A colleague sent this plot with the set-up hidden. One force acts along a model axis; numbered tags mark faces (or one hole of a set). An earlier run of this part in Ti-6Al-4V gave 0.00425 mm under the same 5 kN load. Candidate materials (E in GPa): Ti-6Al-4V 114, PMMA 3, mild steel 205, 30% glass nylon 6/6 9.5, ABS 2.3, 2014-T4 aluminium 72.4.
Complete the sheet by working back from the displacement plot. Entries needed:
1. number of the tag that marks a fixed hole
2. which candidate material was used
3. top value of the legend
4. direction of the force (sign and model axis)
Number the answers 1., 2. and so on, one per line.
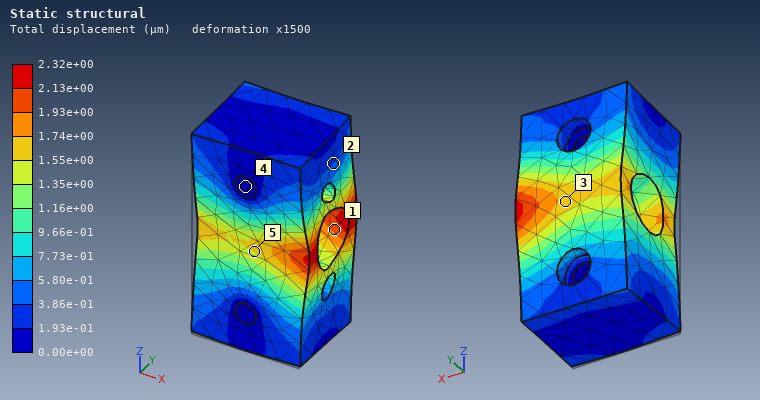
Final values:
1. 4
2. mild steel
3. 2.32e+00 µm
4. +Y
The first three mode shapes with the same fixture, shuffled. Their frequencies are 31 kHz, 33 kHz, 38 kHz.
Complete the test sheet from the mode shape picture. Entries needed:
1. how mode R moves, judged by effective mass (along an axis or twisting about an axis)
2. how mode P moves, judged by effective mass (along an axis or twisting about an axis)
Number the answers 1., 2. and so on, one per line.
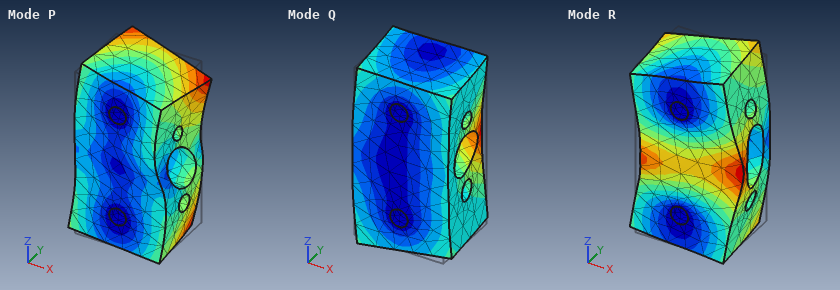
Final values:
1. twisting about Z
2. twisting about Y
